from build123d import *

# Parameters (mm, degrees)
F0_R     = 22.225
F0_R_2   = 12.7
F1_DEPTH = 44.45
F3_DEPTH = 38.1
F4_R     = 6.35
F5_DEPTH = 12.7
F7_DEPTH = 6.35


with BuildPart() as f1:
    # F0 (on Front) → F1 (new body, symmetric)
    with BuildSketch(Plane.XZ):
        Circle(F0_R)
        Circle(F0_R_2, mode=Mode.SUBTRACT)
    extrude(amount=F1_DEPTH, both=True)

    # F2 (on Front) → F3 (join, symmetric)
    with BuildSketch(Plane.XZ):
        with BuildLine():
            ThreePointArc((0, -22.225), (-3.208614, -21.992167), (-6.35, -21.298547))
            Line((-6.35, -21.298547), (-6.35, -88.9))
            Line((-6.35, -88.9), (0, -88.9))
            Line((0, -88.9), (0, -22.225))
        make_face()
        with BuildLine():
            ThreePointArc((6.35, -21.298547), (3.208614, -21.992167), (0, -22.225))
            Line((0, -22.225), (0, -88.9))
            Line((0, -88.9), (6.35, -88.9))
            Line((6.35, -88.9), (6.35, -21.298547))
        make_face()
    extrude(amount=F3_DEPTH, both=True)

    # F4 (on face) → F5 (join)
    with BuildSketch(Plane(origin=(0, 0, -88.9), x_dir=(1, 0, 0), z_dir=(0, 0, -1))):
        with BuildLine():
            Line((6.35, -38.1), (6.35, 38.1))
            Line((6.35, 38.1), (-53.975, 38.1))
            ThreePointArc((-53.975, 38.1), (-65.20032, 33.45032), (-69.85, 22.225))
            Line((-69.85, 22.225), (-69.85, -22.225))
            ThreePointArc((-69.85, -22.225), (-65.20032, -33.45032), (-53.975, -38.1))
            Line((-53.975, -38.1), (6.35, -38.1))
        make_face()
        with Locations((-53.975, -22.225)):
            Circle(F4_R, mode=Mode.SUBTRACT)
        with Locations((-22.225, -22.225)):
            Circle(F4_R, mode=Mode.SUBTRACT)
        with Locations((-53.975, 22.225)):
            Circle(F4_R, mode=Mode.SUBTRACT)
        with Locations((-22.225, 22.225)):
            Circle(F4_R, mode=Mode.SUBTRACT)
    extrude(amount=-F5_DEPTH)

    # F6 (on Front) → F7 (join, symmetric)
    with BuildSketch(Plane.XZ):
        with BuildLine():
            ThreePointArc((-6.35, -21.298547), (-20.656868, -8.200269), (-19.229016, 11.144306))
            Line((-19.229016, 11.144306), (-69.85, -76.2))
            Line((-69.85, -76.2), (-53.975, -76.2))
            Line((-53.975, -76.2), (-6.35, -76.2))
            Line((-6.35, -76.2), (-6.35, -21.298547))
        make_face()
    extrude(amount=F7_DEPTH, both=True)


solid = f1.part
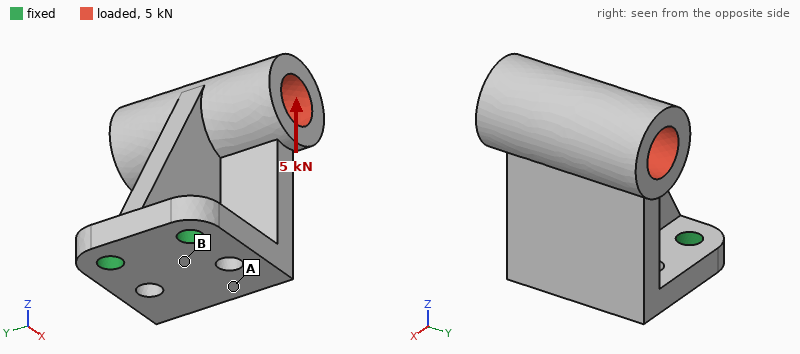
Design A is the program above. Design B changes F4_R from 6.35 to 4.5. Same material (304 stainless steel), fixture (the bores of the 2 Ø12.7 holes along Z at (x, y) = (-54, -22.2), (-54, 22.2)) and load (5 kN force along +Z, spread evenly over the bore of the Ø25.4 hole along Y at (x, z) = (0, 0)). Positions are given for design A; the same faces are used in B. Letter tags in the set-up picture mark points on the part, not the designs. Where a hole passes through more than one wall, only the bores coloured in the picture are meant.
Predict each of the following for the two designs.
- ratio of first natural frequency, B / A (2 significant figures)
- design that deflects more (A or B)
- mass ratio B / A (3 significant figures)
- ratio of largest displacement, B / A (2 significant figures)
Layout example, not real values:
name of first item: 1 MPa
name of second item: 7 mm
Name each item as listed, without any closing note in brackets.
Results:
ratio of first natural frequency, B / A: 0.90
design that deflects more: B
mass ratio B / A: 1.01
ratio of largest displacement, B / A: 1.2
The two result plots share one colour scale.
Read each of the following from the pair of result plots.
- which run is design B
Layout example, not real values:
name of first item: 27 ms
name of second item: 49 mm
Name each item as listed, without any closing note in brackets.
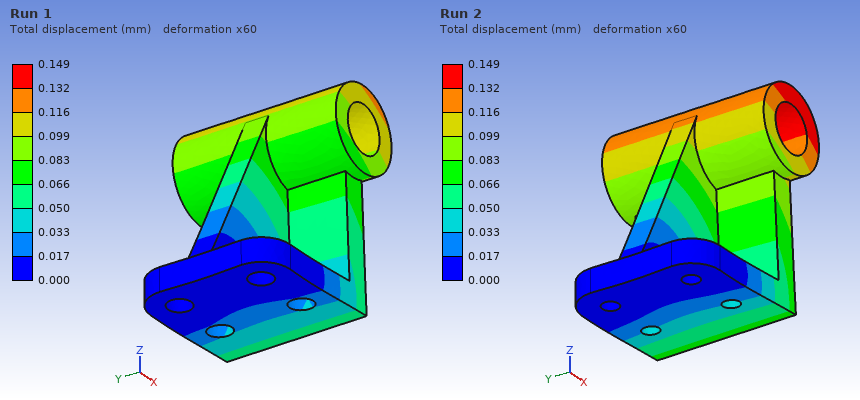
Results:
which run is design B: Run 2
